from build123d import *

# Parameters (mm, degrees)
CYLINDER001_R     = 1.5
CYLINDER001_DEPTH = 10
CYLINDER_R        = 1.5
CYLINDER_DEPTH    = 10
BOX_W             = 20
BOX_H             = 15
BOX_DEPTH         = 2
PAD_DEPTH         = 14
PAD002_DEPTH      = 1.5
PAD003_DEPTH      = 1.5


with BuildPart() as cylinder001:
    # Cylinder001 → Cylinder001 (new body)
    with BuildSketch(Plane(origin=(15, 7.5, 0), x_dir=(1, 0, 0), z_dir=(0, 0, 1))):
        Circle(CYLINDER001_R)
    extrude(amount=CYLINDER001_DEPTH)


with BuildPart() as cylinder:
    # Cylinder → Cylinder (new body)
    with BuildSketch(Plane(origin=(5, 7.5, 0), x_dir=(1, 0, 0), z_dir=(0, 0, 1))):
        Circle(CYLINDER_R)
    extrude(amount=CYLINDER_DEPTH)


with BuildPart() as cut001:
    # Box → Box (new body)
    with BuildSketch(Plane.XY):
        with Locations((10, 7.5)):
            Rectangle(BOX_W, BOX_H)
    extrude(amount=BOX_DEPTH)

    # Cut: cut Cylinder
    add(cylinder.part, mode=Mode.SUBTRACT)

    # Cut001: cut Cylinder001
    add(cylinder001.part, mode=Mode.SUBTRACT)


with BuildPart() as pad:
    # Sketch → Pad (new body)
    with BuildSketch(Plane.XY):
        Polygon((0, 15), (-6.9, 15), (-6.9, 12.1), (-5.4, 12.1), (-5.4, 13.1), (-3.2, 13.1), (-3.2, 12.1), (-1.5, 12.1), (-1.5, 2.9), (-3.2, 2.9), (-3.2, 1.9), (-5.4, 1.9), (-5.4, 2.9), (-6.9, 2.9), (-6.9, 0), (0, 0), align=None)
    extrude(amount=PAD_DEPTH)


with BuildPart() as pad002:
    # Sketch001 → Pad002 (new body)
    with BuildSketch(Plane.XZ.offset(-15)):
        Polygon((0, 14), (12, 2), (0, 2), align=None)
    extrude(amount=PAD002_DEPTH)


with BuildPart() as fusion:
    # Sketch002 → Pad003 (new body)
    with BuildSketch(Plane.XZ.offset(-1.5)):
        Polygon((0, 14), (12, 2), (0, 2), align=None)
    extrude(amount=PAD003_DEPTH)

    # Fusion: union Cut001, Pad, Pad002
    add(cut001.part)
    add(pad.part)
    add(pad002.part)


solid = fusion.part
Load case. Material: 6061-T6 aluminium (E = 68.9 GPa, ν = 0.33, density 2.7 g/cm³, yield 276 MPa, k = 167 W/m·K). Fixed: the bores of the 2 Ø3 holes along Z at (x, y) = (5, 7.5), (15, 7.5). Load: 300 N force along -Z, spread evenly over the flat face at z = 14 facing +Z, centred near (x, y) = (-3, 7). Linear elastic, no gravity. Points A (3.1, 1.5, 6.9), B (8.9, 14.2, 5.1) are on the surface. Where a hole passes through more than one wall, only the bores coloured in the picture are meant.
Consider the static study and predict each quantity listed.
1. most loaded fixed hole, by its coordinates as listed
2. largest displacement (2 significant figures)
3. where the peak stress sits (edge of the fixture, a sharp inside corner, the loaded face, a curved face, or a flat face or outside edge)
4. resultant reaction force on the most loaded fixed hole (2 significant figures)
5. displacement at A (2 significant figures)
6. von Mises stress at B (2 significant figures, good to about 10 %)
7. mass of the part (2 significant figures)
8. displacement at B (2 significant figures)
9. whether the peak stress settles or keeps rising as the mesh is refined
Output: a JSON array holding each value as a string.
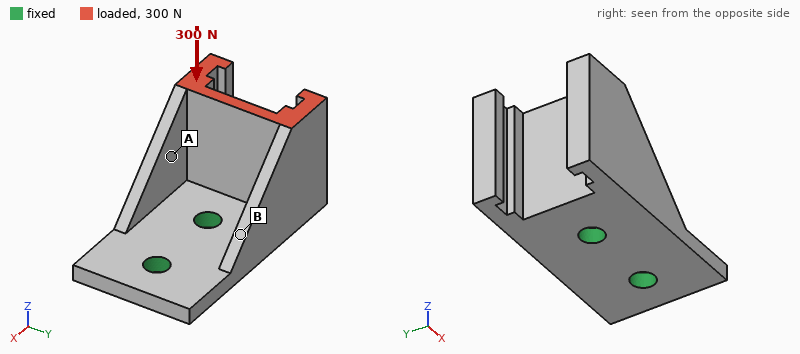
["(5, 7.5)", "57 µm", "edge of the fixture", "420 N", "20 µm", "38 MPa", "4.0 g", "10 µm", "keeps rising"]
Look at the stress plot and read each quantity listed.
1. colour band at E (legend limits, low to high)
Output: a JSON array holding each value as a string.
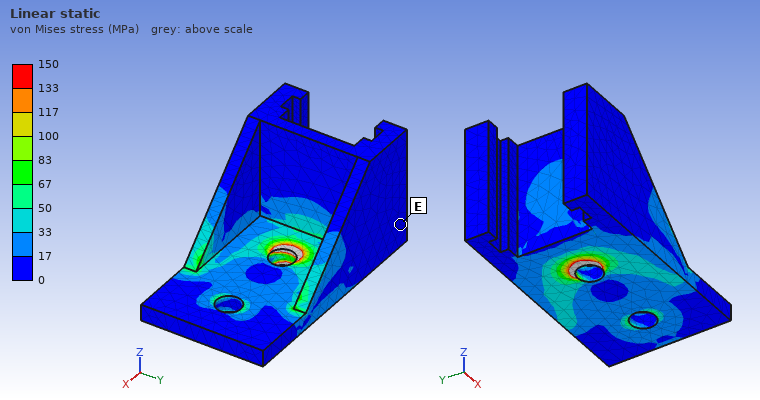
["0 to 17 MPa"]
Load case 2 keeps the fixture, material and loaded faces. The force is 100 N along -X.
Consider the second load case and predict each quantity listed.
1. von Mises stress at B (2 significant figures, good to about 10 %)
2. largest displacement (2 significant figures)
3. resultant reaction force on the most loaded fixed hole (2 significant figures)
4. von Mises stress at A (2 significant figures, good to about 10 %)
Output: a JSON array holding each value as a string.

["30 MPa", "34 µm", "110 N", "14 MPa"]
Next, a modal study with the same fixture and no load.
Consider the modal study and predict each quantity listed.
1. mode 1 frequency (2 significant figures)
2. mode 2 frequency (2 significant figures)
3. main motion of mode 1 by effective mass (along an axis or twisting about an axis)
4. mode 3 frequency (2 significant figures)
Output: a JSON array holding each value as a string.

["6400 Hz", "8600 Hz", "along Y", "17 kHz"]
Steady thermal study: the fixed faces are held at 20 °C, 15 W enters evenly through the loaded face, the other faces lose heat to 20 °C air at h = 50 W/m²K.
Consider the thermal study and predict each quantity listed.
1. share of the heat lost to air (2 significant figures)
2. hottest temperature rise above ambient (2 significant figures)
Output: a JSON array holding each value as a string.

["8.2 %", "33 K"]
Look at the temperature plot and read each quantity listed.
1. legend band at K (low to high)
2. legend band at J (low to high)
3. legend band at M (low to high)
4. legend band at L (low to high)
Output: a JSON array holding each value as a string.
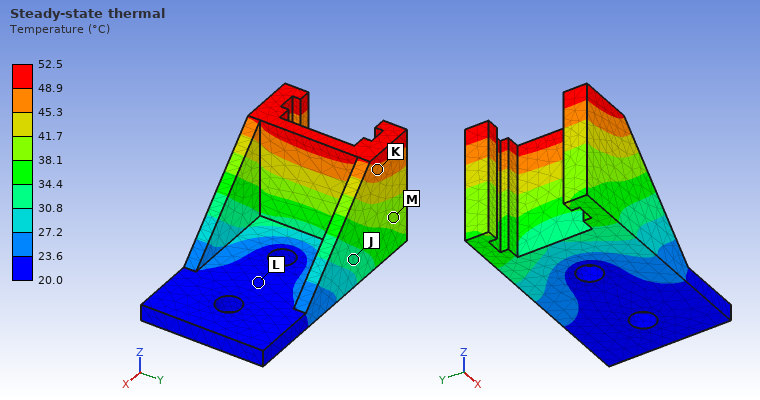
["45.3 to 48.9 °C", "30.8 to 34.4 °C", "38.1 to 41.7 °C", "20.0 to 23.6 °C"]
